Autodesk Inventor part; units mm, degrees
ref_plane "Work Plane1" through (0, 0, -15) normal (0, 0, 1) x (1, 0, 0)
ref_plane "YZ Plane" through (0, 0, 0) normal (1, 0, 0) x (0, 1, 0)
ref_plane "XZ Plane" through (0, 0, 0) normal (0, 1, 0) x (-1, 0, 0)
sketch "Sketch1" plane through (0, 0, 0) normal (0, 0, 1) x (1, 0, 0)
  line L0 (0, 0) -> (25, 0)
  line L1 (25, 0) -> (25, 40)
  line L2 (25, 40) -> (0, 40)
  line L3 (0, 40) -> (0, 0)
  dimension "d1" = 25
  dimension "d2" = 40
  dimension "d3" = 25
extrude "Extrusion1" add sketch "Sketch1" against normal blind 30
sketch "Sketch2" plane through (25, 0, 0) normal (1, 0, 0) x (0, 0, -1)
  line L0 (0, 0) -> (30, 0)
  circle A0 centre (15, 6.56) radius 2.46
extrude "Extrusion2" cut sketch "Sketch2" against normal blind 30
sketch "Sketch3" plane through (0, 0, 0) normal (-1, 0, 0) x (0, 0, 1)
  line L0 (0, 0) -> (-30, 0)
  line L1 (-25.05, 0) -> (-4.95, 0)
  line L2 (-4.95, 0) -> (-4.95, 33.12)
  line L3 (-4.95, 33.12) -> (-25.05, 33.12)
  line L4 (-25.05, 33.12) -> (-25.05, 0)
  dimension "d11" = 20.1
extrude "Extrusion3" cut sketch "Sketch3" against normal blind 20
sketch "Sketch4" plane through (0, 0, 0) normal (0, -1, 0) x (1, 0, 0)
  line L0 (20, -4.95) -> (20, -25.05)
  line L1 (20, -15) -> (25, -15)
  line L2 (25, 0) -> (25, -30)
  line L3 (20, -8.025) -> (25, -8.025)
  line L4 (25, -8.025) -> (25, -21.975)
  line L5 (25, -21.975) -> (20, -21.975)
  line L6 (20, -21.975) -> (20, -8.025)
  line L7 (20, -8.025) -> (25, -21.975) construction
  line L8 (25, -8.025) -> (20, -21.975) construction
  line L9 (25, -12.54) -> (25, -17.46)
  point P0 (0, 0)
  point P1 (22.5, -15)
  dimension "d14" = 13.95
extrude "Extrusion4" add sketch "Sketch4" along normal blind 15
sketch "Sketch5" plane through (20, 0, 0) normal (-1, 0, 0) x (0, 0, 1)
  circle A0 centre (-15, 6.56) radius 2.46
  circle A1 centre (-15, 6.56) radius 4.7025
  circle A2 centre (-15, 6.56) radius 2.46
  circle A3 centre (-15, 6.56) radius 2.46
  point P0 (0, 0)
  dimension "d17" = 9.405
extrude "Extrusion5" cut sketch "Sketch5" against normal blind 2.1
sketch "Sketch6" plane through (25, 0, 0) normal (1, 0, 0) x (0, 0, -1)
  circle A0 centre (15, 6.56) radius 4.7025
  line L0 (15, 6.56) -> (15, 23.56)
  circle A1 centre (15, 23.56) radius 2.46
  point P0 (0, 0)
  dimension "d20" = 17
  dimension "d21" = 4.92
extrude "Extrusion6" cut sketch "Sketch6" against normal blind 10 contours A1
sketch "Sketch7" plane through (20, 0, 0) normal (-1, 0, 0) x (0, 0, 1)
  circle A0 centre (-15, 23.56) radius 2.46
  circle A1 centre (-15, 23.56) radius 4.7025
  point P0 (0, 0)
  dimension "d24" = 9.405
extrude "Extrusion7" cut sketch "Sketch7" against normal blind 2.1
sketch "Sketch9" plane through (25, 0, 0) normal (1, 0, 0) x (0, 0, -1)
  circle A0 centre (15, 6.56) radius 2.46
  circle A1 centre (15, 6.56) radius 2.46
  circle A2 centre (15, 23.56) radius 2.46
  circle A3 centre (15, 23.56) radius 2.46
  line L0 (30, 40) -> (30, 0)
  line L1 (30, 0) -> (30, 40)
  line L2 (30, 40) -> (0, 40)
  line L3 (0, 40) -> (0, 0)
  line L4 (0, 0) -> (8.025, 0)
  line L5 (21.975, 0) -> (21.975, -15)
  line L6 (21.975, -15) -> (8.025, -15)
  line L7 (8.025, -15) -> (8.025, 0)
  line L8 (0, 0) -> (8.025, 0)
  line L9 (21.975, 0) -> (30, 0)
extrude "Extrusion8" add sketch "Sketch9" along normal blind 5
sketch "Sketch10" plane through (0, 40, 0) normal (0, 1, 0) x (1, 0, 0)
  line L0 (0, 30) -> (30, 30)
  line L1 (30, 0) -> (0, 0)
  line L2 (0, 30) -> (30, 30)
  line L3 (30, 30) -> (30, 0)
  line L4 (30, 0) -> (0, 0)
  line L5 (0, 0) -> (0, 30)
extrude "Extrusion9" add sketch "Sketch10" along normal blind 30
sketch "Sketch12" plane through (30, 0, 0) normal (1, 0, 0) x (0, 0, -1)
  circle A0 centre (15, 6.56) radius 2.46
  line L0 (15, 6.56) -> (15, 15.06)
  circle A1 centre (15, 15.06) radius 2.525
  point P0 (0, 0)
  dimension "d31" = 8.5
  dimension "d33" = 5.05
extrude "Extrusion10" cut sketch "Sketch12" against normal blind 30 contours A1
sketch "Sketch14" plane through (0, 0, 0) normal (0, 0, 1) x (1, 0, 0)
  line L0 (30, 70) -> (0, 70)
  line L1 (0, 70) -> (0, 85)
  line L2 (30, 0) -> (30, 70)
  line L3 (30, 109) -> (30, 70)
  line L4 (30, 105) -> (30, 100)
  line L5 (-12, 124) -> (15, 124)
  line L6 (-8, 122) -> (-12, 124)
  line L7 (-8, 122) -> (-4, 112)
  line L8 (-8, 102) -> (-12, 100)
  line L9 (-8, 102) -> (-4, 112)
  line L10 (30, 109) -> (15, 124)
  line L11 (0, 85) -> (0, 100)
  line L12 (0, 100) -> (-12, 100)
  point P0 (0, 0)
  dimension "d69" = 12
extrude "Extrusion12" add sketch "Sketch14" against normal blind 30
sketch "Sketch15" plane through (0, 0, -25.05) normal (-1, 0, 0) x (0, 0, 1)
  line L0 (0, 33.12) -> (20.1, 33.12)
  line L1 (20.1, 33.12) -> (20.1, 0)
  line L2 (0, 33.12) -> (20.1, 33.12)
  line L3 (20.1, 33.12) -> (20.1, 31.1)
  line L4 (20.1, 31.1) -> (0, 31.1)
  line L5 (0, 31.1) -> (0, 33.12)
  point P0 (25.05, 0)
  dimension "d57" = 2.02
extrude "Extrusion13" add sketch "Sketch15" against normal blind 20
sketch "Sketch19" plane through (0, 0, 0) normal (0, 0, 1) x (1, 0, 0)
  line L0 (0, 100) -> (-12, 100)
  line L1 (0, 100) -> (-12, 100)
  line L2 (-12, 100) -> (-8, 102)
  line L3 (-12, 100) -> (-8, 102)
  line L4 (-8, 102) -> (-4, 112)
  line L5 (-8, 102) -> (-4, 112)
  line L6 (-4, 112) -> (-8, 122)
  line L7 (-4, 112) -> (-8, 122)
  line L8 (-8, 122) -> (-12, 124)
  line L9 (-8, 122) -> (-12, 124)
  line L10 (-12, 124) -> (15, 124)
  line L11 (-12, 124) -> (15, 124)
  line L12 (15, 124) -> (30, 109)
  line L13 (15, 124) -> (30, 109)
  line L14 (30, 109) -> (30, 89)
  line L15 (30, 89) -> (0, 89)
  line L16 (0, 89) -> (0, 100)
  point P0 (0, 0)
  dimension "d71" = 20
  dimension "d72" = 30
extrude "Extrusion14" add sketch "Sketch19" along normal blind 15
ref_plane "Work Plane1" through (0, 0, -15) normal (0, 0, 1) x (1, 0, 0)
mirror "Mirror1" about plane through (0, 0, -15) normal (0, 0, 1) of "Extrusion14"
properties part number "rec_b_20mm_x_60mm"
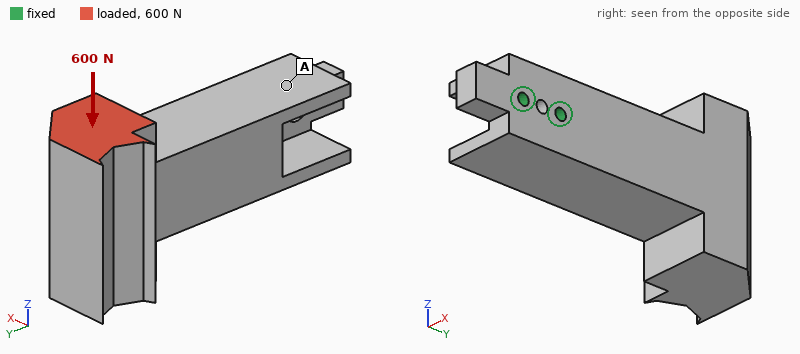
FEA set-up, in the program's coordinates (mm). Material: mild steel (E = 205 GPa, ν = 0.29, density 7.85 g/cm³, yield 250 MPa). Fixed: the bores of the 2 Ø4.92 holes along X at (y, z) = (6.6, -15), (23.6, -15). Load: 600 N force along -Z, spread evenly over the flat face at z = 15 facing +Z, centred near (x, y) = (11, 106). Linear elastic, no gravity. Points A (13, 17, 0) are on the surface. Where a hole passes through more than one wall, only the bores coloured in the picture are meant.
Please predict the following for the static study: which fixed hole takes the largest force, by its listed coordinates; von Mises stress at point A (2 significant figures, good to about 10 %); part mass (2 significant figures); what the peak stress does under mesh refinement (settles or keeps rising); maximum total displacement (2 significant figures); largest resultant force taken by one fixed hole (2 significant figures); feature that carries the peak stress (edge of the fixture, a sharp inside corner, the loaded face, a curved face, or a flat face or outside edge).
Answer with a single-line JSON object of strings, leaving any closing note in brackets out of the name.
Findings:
{"which fixed hole takes the largest force, by its listed coordinates": "(23.6, -15)", "von Mises stress at point A": "10 MPa", "part mass": "1.1 kg", "what the peak stress does under mesh refinement": "keeps rising", "maximum total displacement": "38 µm", "largest resultant force taken by one fixed hole": "2.7 kN", "feature that carries the peak stress": "edge of the fixture"}
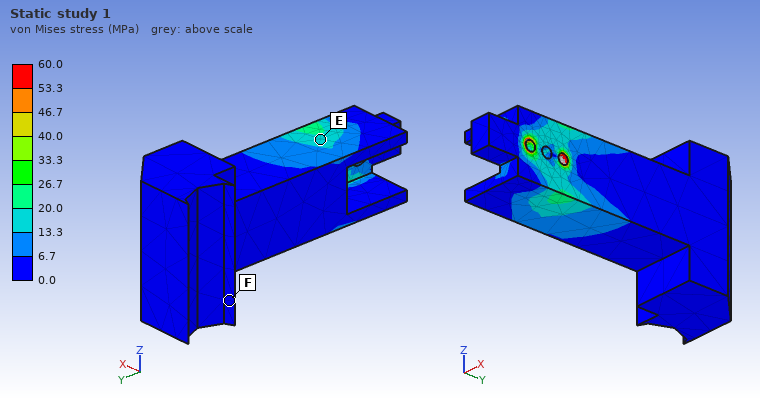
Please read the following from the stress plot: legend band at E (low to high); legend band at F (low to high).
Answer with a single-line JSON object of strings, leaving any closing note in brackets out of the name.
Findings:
{"legend band at E": "13.3 to 20.0 MPa", "legend band at F": "0.0 to 6.7 MPa"}
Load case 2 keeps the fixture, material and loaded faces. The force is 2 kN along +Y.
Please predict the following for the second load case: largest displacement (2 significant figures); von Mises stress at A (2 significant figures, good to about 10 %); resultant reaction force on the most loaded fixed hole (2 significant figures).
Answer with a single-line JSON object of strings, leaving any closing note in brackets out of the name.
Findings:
{"largest displacement": "60 µm", "von Mises stress at A": "19 MPa", "resultant reaction force on the most loaded fixed hole": "3.1 kN"}
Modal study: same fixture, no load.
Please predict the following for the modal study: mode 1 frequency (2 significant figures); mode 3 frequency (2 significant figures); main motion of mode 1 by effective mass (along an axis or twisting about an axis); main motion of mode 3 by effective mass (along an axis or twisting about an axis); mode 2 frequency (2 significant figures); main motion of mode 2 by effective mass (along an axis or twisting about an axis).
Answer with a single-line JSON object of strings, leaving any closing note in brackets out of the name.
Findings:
{"mode 1 frequency": "800 Hz", "mode 3 frequency": "2100 Hz", "main motion of mode 1 by effective mass": "along X", "main motion of mode 3 by effective mass": "twisting about Y", "mode 2 frequency": "920 Hz", "main motion of mode 2 by effective mass": "along Z"}
